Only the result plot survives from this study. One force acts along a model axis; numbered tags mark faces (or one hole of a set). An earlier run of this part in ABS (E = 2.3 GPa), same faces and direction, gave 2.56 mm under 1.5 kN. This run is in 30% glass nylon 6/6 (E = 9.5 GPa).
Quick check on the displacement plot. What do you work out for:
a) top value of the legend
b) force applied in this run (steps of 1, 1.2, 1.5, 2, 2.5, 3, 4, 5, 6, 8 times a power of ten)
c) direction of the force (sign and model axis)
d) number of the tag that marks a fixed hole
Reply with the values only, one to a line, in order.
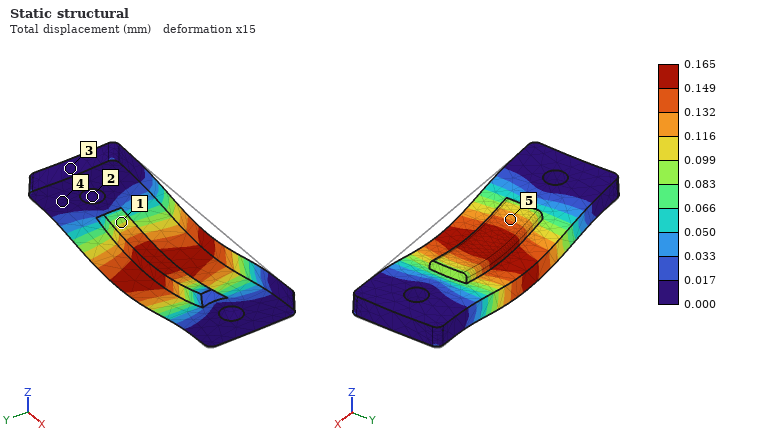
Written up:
0.165 mm
400 N
-Z
2
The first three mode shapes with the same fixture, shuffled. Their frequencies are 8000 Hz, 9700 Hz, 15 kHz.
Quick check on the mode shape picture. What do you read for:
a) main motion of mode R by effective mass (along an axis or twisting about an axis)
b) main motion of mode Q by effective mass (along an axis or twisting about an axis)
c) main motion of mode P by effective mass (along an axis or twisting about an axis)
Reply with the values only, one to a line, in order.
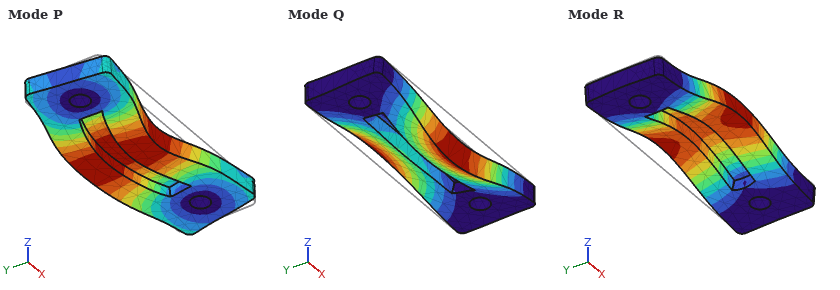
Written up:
along Z
twisting about X
along Y
